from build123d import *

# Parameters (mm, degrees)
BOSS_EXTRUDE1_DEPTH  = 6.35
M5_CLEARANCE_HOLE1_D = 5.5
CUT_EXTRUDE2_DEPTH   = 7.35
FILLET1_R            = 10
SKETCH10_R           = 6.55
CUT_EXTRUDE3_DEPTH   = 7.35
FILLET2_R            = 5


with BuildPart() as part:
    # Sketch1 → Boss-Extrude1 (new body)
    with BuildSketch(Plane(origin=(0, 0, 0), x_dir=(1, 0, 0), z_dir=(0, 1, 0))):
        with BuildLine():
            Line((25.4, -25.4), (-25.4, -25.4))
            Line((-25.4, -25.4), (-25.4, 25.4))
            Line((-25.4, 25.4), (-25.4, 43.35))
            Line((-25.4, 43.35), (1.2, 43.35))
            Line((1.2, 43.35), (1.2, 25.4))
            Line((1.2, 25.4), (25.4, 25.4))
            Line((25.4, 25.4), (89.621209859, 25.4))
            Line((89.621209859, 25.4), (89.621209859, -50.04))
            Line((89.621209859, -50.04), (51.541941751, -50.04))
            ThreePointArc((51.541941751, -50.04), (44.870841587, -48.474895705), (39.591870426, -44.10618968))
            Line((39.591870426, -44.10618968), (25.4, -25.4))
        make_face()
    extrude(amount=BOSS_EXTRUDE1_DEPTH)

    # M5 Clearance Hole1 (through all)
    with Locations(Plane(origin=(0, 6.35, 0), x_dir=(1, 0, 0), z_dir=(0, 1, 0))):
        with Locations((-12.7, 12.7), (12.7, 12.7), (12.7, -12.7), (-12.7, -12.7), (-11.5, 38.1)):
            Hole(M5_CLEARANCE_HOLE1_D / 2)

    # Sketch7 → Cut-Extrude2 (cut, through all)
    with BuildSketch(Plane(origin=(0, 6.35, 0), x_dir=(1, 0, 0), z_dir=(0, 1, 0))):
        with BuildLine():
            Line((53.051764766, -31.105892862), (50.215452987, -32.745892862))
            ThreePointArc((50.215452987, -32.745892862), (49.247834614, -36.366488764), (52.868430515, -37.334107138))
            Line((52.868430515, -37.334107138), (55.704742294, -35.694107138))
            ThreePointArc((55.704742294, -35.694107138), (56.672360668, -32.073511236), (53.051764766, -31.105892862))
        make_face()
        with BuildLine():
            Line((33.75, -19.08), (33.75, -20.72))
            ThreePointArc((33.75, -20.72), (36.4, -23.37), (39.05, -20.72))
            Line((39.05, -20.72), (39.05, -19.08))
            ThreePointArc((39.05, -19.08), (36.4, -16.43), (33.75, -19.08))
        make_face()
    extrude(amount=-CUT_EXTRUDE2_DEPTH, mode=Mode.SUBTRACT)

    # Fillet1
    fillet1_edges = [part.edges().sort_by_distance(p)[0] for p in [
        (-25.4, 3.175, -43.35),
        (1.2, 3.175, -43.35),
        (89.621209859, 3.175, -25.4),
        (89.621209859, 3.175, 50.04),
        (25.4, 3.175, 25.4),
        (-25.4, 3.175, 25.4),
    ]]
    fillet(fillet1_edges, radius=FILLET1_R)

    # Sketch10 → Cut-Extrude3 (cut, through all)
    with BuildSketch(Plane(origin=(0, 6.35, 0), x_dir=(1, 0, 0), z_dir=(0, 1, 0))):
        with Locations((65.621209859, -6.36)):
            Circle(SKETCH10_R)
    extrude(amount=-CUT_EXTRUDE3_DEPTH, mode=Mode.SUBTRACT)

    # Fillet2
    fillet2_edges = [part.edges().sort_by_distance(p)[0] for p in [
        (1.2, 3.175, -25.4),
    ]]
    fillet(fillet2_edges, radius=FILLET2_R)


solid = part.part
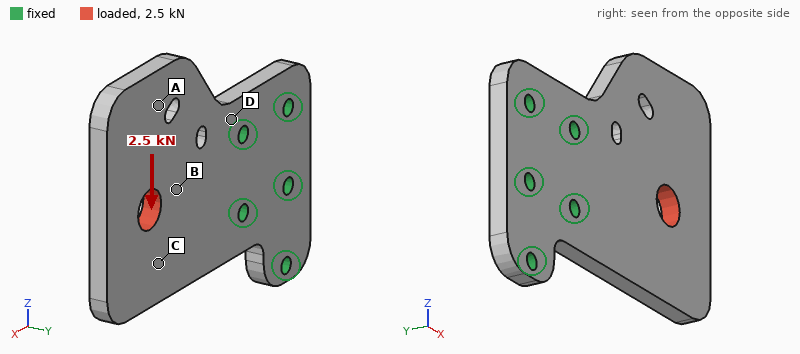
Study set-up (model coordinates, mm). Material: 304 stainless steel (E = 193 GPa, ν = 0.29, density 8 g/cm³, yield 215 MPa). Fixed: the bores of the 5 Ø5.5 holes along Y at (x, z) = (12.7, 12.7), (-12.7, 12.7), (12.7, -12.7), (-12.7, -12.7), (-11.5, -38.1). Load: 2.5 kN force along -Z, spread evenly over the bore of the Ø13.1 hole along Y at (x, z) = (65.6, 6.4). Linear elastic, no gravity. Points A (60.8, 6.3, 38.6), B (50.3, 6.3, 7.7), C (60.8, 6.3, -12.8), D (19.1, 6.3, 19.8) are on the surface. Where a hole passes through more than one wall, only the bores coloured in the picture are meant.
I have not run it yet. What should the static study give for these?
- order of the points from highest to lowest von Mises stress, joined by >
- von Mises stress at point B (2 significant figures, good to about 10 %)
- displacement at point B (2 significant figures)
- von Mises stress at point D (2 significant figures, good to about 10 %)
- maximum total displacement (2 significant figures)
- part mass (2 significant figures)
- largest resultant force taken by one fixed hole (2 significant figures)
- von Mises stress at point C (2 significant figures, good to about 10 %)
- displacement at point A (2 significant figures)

D > B > C > A
19 MPa
12 µm
26 MPa
30 µm
370 g
3.6 kN
12 MPa
21 µm
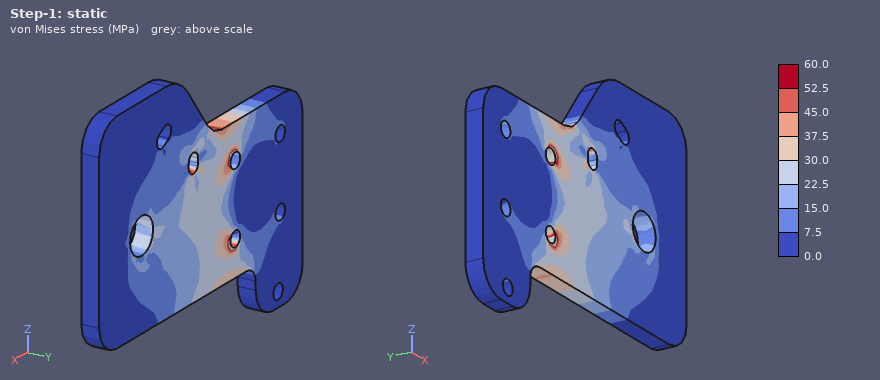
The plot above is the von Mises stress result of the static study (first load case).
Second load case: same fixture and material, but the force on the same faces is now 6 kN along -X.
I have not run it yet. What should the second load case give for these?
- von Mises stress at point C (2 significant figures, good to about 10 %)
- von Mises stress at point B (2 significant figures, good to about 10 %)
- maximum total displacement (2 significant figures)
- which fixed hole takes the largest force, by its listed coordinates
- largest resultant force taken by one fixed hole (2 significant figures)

11 MPa
28 MPa
10 µm
(12.7, 12.7)
3.5 kN
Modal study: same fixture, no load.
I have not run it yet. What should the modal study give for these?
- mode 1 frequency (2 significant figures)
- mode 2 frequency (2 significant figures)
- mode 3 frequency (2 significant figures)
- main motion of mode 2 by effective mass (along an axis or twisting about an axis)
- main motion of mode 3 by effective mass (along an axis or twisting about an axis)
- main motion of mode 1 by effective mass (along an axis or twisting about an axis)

720 Hz
1700 Hz
3900 Hz
twisting about X
along Z
along Y
